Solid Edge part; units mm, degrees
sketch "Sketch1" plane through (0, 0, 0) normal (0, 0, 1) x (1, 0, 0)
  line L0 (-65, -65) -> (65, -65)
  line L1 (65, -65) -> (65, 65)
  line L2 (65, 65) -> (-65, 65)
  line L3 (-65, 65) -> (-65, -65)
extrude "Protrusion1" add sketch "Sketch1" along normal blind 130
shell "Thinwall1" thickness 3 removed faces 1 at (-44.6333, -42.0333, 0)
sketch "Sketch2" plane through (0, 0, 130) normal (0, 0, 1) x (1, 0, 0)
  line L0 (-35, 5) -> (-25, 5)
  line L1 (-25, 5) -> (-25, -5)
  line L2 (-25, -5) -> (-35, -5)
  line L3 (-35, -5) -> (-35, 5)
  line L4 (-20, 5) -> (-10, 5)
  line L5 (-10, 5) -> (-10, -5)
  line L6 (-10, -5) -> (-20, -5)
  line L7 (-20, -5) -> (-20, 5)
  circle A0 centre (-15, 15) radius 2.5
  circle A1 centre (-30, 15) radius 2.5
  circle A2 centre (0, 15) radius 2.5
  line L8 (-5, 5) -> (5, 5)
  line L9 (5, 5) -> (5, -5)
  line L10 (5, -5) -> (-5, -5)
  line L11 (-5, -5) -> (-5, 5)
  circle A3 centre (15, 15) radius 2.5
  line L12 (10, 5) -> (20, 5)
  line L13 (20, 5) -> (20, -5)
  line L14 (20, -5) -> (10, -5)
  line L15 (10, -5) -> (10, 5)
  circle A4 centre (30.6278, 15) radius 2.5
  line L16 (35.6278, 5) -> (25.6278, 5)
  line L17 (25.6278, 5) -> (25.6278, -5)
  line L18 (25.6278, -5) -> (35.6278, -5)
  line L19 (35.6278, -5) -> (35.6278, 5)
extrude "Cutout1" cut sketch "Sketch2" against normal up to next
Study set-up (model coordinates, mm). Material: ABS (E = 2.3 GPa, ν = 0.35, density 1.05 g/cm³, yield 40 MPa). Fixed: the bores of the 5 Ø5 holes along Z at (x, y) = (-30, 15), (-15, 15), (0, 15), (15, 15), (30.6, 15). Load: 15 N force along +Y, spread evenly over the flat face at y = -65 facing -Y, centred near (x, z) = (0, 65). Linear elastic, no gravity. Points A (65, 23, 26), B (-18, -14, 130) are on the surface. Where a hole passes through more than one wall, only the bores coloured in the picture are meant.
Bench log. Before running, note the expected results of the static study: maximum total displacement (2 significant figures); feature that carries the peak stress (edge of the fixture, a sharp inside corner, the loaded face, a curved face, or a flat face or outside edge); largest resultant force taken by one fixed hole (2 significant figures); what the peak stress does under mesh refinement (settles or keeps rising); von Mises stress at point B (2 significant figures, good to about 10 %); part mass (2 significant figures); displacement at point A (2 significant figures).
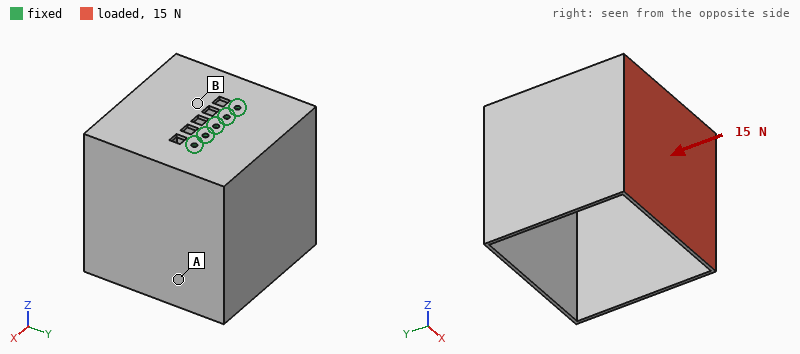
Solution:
2.6 mm
edge of the fixture
6.5 N
keeps rising
0.71 MPa
250 g
1.6 mm
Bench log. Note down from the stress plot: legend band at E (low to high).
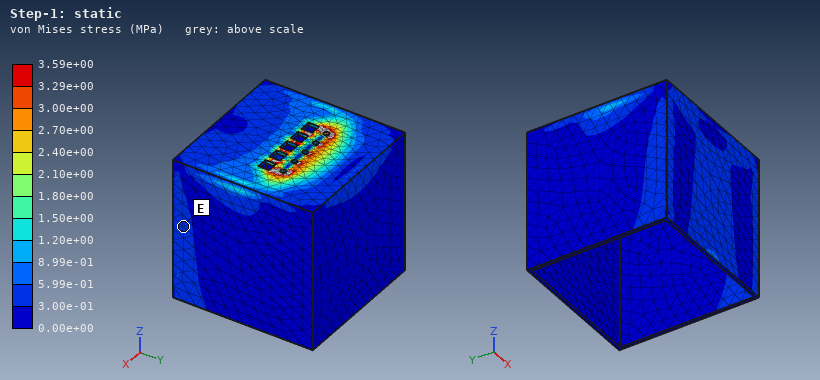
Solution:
3.00e-01 to 5.99e-01 MPa
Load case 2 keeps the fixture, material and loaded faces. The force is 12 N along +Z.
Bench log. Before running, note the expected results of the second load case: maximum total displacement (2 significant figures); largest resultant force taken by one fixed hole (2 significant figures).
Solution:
2.6 mm
9.7 N
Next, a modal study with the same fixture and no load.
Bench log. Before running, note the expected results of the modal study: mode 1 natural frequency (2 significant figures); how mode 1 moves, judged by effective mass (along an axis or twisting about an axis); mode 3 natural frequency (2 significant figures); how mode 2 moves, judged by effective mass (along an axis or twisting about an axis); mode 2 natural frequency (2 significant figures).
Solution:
29 Hz
along Y
90 Hz
along X
62 Hz
